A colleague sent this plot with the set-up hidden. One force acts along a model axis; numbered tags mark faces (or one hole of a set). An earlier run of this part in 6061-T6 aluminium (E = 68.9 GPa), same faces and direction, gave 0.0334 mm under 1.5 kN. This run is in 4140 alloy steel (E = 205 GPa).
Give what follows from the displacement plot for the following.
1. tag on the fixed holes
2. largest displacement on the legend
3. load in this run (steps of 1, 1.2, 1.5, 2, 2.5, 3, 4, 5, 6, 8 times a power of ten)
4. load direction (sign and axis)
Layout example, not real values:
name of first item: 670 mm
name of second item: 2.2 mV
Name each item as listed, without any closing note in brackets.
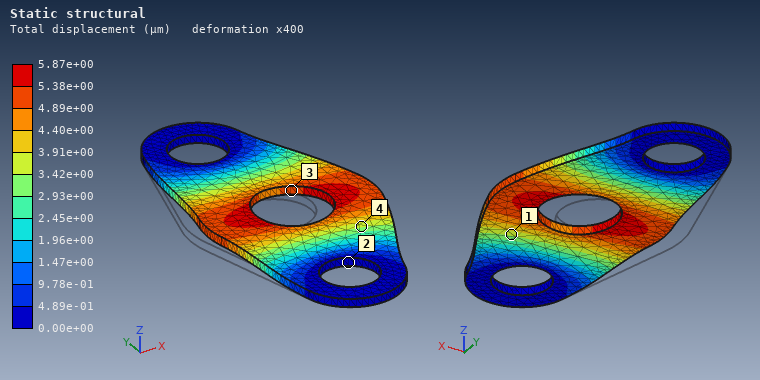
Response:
tag on the fixed holes: 2
largest displacement on the legend: 5.87e+00 µm
load in this run: 800 N
load direction: +X
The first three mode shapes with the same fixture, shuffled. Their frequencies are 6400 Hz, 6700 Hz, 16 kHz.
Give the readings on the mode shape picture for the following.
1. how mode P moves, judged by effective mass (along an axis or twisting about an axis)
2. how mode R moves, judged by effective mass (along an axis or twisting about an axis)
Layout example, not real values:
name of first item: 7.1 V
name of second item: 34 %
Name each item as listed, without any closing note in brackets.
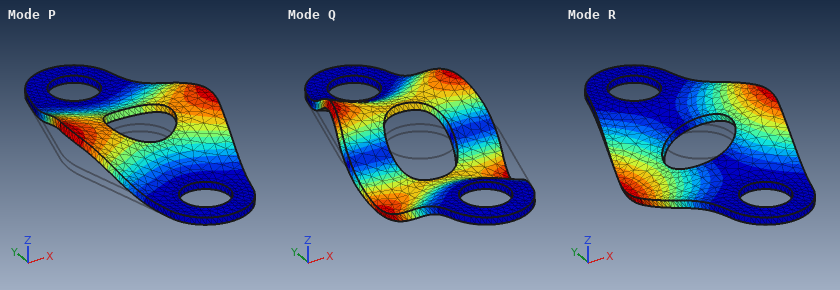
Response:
how mode P moves, judged by effective mass: along Z
how mode R moves, judged by effective mass: twisting about Y
